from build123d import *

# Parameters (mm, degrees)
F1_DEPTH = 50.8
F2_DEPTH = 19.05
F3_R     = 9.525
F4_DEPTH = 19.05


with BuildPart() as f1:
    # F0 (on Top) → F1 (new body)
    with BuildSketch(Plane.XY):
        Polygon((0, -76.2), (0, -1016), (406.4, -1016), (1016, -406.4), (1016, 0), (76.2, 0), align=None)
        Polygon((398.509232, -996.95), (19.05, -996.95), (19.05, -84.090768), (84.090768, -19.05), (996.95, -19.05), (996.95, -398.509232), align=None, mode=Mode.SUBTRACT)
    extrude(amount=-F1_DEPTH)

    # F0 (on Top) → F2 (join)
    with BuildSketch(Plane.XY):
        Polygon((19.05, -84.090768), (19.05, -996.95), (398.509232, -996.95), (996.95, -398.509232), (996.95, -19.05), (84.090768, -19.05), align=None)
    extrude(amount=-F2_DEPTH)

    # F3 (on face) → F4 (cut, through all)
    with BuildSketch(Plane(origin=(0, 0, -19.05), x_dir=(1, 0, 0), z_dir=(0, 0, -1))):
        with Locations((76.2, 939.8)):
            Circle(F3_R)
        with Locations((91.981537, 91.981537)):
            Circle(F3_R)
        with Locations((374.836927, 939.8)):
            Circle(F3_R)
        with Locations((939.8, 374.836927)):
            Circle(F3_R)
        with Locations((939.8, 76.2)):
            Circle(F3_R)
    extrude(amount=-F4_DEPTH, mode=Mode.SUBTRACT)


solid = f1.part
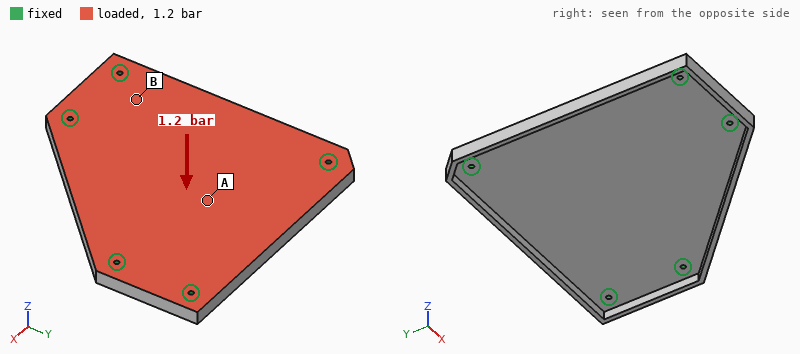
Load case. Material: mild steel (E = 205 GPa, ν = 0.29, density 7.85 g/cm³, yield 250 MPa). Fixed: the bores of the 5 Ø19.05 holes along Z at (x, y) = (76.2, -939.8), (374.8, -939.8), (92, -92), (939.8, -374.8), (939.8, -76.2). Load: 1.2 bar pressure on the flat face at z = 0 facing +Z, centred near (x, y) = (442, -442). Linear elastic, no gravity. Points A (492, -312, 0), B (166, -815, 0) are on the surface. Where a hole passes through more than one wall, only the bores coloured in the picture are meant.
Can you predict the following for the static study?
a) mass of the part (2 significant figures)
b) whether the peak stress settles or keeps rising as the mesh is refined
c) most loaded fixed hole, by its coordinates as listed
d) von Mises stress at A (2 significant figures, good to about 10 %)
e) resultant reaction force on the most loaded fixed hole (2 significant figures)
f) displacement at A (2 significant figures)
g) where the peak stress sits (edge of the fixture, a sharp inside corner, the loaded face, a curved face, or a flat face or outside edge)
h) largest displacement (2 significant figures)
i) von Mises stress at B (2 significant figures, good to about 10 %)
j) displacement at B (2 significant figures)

140 kg
keeps rising
(92, -92)
53 MPa
30 kN
1.7 mm
edge of the fixture
1.8 mm
18 MPa
0.43 mm
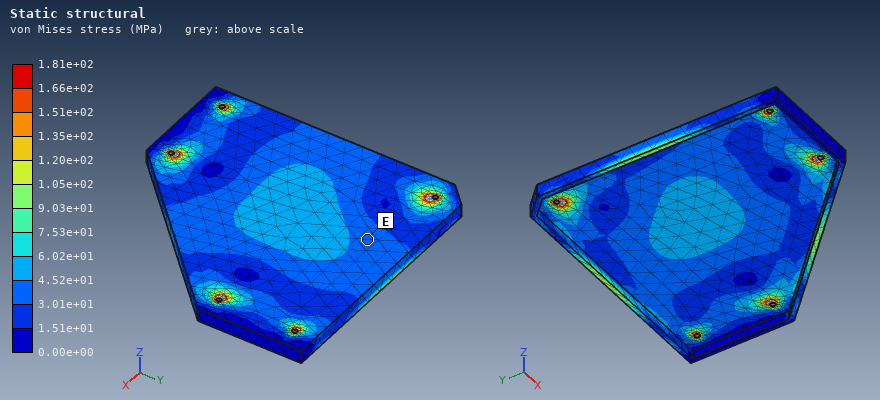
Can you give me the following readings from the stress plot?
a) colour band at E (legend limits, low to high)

3.01e+01 to 4.52e+01 MPa
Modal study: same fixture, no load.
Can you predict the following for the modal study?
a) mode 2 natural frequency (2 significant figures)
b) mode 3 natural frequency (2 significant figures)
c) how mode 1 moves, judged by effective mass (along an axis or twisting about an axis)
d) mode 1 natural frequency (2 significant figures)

190 Hz
240 Hz
along Z
130 Hz
